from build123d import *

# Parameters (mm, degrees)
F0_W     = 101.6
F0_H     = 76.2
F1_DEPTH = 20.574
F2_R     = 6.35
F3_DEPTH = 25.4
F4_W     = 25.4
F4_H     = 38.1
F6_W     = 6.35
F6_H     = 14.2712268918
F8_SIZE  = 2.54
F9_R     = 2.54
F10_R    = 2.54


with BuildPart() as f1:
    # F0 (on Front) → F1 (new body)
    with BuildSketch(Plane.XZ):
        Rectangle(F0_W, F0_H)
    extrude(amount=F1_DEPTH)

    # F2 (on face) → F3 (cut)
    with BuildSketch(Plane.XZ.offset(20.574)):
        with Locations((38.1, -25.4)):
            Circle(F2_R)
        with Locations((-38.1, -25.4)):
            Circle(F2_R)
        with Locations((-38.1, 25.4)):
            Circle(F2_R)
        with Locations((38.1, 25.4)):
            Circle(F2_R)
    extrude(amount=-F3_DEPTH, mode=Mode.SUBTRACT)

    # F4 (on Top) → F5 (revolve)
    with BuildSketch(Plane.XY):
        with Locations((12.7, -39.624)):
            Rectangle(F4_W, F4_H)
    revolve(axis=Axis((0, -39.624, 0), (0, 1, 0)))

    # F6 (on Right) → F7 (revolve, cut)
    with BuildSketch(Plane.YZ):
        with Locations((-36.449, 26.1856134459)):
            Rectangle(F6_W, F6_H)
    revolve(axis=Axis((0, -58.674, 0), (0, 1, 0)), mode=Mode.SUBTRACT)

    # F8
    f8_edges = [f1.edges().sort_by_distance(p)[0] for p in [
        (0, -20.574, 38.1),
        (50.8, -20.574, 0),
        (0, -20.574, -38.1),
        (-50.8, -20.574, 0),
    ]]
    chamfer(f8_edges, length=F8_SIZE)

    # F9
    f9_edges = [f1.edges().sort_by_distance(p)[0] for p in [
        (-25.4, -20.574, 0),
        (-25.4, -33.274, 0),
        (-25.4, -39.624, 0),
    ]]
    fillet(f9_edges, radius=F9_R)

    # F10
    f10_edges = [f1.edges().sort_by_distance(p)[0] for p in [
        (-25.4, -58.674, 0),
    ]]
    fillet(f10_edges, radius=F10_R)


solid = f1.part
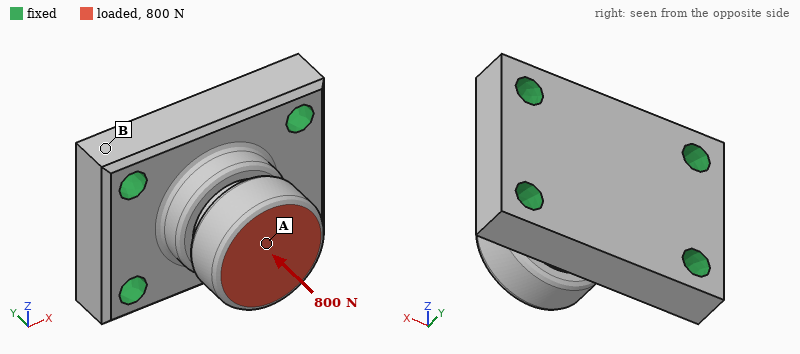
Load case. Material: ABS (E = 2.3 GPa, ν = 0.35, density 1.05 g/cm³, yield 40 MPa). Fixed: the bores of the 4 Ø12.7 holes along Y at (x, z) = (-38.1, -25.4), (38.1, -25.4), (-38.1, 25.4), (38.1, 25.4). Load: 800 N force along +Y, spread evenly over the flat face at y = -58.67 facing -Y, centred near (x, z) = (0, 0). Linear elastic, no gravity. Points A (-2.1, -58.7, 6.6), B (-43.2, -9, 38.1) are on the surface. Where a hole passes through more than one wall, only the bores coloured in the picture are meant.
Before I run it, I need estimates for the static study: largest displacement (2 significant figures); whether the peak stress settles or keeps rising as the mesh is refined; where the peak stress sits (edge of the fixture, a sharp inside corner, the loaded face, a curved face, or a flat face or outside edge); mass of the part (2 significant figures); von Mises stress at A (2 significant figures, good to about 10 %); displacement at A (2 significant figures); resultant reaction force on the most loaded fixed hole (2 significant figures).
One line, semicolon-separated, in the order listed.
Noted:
23 µm; keeps rising; edge of the fixture; 230 g; 0.59 MPa; 22 µm; 210 N
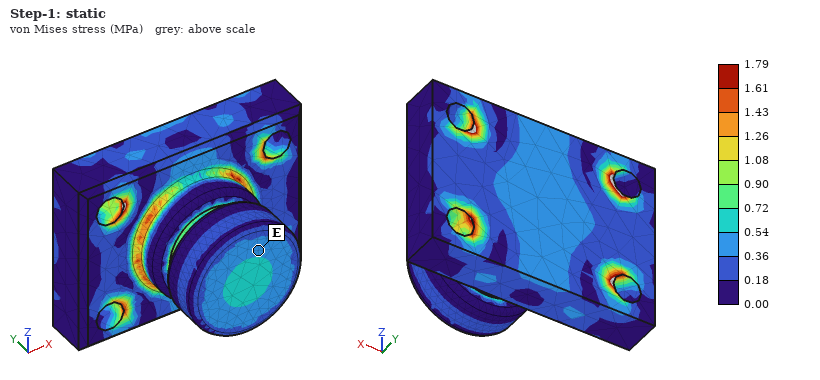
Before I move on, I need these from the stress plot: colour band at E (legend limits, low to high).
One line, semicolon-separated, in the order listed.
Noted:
0.36 to 0.54 MPa
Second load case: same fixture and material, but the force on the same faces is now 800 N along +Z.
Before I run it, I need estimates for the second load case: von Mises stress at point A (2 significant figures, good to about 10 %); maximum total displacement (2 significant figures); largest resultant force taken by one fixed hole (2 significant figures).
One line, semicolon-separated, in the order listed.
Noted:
0.97 MPa; 0.14 mm; 440 N
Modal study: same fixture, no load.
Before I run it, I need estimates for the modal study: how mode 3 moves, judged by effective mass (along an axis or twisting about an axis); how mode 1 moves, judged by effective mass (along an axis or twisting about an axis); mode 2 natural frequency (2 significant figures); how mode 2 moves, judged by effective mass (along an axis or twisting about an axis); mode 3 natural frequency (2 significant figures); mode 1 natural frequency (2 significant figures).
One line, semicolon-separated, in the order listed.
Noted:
along Y; along Z; 2600 Hz; along X; 3100 Hz; 2200 Hz
